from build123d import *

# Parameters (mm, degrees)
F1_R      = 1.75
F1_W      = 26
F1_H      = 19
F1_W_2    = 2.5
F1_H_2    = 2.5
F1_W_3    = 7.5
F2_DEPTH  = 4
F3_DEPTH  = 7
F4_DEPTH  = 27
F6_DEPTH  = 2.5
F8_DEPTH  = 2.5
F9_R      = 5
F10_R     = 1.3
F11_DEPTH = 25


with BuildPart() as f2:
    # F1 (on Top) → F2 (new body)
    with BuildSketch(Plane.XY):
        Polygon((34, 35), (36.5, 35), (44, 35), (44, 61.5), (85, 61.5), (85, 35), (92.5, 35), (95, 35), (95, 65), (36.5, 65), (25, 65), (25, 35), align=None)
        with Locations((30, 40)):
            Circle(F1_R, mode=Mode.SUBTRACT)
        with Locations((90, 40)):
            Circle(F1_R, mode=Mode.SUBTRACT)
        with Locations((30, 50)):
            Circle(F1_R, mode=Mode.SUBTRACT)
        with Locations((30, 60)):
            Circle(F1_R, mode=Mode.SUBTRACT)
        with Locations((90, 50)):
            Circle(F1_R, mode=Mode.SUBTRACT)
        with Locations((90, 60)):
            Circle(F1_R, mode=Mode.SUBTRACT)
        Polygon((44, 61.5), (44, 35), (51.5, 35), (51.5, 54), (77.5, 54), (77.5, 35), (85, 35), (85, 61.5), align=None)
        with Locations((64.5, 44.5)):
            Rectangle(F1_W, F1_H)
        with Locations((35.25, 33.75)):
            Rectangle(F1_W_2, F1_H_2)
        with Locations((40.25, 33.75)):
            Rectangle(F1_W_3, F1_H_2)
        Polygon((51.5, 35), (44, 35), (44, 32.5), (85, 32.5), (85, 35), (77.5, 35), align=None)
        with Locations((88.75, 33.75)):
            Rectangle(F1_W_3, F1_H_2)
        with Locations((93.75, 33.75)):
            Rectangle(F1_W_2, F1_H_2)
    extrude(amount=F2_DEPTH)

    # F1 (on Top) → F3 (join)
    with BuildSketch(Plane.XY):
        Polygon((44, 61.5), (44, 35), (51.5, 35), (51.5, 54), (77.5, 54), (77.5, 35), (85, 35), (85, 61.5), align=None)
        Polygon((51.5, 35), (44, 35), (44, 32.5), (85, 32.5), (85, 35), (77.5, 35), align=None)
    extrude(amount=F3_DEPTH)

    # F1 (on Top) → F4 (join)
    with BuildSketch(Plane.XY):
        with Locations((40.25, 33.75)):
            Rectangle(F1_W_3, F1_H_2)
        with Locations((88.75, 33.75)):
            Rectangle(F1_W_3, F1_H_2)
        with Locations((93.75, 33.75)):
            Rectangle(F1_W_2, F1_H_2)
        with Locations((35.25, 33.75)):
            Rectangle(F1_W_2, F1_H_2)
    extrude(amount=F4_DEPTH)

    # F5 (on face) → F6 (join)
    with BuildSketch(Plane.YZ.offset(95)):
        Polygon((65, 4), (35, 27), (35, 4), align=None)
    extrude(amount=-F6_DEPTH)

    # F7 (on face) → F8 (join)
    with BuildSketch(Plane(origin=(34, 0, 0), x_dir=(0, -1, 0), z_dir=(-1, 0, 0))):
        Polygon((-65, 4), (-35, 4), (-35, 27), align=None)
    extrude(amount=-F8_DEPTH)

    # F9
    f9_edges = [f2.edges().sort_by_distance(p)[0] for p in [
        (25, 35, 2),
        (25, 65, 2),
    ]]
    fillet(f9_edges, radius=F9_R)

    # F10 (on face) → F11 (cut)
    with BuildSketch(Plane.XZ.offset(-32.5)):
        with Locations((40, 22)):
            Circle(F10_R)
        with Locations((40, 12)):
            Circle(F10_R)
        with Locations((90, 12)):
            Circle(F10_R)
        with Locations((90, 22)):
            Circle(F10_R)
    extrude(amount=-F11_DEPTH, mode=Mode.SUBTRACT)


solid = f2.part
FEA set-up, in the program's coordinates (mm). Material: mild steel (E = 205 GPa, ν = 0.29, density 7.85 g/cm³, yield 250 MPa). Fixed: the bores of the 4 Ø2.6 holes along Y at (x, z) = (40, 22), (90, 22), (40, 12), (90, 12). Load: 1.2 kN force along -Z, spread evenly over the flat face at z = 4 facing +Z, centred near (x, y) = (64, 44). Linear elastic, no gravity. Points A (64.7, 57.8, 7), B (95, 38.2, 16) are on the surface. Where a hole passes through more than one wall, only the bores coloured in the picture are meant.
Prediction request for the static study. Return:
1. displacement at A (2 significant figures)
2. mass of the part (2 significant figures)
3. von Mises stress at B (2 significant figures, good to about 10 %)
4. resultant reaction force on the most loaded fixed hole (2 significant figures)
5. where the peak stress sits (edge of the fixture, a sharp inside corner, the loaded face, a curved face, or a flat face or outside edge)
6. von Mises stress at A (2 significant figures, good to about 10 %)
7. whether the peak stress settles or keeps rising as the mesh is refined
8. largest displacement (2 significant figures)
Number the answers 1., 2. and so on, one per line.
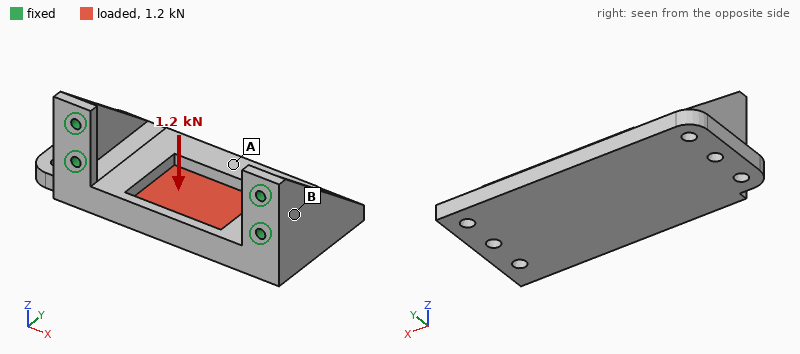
1. 45 µm
2. 110 g
3. 18 MPa
4. 860 N
5. edge of the fixture
6. 57 MPa
7. keeps rising
8. 55 µm
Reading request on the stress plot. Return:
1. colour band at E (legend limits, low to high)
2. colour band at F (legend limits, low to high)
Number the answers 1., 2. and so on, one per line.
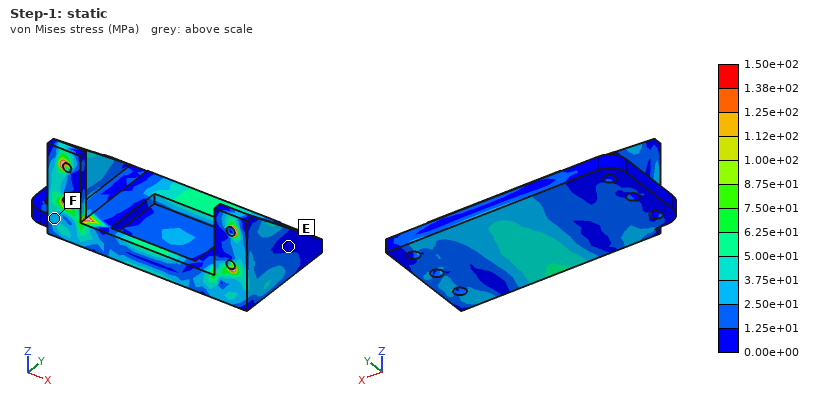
1. 0.00e+00 to 1.25e+01 MPa
2. 2.50e+01 to 3.75e+01 MPa
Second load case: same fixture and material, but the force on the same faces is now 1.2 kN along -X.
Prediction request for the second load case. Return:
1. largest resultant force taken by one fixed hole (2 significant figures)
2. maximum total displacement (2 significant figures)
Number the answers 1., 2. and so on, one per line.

1. 820 N
2. 16 µm
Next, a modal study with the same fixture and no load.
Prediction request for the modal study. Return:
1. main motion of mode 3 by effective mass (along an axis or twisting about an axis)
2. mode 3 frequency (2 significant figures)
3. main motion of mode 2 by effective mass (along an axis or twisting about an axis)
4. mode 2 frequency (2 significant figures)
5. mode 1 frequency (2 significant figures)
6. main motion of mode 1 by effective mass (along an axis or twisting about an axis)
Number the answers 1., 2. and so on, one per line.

1. along Y
2. 6800 Hz
3. along X
4. 4400 Hz
5. 2800 Hz
6. along Z
